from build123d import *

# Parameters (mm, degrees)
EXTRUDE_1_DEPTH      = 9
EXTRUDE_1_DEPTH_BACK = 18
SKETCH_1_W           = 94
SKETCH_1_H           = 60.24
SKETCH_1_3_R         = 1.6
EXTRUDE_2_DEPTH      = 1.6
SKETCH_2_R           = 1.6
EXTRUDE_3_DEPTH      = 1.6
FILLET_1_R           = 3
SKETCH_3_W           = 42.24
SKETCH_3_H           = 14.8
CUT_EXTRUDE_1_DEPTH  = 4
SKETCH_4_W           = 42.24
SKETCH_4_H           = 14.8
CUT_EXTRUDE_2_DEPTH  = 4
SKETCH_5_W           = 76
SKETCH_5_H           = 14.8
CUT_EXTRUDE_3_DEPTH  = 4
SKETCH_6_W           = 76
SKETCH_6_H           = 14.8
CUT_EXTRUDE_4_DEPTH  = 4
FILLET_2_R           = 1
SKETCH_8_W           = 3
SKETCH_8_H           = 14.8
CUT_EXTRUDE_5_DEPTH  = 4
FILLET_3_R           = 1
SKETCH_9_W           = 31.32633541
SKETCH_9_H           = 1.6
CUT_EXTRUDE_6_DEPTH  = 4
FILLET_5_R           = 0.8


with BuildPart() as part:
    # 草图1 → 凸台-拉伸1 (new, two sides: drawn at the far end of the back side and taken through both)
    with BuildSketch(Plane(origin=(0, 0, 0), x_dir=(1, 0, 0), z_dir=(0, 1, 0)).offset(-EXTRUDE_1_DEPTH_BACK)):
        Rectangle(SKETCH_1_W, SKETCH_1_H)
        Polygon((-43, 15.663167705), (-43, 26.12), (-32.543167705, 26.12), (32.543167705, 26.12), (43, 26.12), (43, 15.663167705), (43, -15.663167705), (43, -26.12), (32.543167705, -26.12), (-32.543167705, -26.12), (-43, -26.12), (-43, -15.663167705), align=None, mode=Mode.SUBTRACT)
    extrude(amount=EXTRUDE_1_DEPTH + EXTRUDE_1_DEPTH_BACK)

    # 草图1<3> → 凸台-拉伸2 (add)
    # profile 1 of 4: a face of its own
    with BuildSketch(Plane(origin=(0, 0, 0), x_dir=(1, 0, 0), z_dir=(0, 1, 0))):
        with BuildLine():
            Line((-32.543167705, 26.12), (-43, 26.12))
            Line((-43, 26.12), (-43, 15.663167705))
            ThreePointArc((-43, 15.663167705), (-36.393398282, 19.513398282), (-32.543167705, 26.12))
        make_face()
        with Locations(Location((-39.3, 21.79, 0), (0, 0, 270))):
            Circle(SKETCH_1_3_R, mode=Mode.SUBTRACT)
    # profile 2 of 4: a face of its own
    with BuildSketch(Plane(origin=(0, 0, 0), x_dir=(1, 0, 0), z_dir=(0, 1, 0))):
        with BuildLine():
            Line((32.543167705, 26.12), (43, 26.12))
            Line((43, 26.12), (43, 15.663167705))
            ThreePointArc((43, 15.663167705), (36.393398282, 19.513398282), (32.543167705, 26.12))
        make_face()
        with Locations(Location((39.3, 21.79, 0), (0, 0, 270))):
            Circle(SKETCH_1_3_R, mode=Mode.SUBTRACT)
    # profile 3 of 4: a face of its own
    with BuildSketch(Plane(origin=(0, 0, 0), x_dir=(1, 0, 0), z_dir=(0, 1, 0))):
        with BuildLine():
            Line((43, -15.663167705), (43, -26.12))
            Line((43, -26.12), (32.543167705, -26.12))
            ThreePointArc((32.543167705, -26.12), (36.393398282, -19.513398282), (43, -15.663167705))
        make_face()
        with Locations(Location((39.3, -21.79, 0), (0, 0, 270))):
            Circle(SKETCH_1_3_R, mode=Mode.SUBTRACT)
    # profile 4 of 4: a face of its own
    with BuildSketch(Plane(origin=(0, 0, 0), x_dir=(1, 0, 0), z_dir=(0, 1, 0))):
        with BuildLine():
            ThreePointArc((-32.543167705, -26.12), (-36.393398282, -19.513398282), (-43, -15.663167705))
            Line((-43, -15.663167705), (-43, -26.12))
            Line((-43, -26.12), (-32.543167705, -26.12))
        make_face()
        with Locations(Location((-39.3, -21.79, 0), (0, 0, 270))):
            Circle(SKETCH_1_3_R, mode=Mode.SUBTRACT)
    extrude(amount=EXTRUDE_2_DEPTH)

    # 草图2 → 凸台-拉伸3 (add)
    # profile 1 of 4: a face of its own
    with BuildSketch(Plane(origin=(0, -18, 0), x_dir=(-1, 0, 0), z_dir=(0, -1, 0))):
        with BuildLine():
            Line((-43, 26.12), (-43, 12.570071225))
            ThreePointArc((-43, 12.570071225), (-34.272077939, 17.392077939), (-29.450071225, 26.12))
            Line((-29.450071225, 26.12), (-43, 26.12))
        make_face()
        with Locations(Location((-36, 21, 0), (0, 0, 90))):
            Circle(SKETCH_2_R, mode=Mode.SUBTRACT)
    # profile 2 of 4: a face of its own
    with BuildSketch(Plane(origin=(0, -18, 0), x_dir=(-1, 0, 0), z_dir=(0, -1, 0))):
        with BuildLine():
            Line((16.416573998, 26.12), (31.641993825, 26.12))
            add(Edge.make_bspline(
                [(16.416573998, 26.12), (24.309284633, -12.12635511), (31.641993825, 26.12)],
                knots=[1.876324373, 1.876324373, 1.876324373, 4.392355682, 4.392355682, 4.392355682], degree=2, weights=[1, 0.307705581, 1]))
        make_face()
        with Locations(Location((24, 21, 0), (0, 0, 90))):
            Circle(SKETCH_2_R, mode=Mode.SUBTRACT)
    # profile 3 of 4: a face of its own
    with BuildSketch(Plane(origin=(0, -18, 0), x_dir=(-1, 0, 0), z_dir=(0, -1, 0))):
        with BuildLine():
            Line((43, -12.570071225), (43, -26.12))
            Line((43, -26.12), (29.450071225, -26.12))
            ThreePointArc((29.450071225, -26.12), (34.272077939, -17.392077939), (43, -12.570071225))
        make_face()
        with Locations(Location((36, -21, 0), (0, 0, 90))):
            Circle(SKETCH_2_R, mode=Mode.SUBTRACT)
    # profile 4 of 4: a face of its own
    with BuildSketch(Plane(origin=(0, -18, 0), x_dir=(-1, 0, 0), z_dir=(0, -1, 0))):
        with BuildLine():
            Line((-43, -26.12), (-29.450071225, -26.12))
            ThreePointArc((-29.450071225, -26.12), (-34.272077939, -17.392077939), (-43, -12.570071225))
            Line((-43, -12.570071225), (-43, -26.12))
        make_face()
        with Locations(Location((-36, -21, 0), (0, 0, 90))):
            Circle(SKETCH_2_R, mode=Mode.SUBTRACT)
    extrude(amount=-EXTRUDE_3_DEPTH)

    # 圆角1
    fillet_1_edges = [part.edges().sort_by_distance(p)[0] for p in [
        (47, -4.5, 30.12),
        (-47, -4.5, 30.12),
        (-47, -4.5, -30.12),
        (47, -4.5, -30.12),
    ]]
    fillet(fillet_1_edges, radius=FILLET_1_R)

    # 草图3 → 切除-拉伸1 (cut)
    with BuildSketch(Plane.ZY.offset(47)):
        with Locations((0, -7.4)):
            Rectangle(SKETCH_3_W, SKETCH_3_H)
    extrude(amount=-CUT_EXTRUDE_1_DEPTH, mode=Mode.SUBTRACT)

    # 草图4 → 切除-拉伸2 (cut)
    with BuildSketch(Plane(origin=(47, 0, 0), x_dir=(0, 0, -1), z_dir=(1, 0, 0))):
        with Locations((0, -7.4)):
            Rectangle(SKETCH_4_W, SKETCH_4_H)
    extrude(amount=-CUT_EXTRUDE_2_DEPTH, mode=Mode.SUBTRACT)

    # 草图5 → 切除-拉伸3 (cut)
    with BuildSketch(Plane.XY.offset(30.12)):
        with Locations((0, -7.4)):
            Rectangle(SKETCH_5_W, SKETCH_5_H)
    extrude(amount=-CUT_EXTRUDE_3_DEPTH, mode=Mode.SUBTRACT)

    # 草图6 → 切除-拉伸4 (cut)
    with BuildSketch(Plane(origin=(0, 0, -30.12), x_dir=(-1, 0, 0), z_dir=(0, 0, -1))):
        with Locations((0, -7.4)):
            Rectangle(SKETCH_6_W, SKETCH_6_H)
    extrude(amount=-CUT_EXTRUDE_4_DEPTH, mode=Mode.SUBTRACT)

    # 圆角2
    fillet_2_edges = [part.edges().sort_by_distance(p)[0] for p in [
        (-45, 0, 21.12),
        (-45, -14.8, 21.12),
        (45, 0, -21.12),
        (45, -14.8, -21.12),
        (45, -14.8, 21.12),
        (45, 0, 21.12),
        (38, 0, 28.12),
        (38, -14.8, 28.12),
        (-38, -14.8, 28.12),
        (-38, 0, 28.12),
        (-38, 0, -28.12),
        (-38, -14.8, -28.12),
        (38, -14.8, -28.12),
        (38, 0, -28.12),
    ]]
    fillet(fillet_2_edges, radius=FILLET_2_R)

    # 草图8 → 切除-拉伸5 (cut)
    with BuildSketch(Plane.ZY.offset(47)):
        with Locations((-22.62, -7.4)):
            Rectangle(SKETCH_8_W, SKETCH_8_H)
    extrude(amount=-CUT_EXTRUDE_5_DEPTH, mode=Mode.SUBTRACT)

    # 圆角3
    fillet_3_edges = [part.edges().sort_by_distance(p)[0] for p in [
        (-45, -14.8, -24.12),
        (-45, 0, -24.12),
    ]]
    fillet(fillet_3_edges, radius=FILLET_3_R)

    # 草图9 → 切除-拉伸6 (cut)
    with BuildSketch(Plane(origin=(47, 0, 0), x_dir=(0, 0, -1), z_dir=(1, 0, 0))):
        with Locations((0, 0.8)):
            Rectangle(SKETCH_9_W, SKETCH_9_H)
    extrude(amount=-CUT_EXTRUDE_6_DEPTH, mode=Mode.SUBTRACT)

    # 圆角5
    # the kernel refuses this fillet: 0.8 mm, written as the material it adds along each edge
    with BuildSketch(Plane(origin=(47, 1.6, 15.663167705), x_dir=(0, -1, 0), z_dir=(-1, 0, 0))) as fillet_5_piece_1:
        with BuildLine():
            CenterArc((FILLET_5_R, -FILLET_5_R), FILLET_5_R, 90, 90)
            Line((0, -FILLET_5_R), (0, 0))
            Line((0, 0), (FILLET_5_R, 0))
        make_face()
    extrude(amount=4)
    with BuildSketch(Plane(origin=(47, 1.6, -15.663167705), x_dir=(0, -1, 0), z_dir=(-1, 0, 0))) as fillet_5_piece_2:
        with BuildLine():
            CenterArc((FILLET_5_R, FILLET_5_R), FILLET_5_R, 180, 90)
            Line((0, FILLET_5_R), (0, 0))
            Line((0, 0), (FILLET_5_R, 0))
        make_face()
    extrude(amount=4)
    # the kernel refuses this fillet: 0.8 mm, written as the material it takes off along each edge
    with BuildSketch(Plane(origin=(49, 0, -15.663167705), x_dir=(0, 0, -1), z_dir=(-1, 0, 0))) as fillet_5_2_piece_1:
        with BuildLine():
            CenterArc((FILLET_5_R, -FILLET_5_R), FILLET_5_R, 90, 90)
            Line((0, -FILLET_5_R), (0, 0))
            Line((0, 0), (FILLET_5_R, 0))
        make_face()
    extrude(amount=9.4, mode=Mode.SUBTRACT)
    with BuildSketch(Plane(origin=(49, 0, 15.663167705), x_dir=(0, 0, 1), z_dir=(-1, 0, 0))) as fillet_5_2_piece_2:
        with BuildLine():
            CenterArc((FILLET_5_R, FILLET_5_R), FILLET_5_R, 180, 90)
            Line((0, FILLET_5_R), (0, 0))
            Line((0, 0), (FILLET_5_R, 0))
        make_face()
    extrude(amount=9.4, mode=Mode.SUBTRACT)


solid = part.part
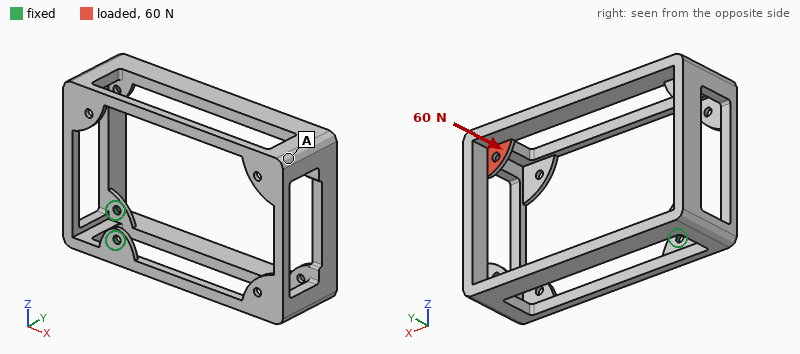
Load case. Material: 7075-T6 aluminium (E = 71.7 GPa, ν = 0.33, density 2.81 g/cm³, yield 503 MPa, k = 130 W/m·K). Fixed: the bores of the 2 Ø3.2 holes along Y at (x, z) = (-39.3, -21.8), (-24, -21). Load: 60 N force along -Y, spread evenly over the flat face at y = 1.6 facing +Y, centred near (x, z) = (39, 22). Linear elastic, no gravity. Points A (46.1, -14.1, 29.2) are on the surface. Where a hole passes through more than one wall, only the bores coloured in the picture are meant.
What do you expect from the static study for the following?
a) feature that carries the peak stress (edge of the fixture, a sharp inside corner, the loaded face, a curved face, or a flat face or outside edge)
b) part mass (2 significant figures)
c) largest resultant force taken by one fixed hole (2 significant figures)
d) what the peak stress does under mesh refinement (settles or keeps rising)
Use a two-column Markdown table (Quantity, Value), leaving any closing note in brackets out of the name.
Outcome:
| Quantity | Value |
|---|---|
| feature that carries the peak stress | edge of the fixture |
| part mass | 51 g |
| largest resultant force taken by one fixed hole | 280 N |
| what the peak stress does under mesh refinement | keeps rising |
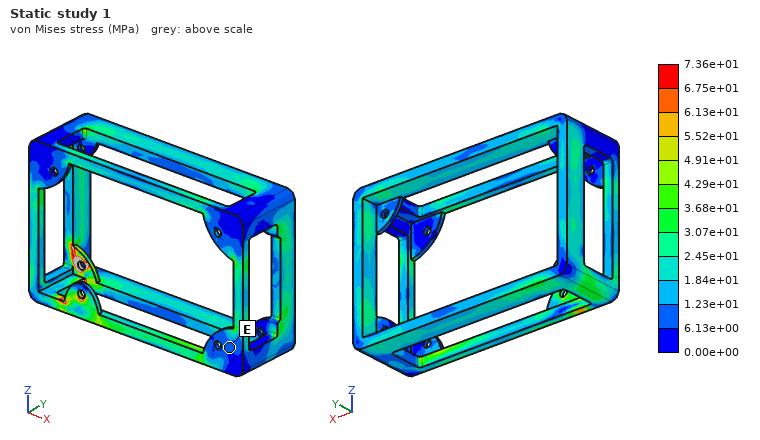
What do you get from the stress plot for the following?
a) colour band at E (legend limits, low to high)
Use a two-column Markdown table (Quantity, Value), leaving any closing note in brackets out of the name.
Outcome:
| Quantity | Value |
|---|---|
| colour band at E | 6.13e+00 to 1.23e+01 MPa |
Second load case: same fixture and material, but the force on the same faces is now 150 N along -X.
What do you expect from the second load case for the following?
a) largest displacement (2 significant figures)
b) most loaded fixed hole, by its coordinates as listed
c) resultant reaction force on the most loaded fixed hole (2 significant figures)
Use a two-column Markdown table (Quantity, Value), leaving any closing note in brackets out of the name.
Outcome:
| Quantity | Value |
|---|---|
| largest displacement | 1.3 mm |
| most loaded fixed hole, by its coordinates as listed | (-39.3, -21.8) |
| resultant reaction force on the most loaded fixed hole | 170 N |
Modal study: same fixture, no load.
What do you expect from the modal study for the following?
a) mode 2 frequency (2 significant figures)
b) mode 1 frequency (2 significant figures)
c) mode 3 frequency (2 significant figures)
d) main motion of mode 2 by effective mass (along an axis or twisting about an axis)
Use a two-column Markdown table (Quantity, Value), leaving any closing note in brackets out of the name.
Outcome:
| Quantity | Value |
|---|---|
| mode 2 frequency | 360 Hz |
| mode 1 frequency | 250 Hz |
| mode 3 frequency | 740 Hz |
| main motion of mode 2 by effective mass | along Y |
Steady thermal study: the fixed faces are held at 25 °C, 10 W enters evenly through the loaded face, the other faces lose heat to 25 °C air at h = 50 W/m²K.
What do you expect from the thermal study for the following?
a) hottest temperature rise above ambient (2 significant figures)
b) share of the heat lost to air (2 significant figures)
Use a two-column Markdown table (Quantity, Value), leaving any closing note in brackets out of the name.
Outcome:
| Quantity | Value |
|---|---|
| hottest temperature rise above ambient | 48 K |
| share of the heat lost to air | 88 % |
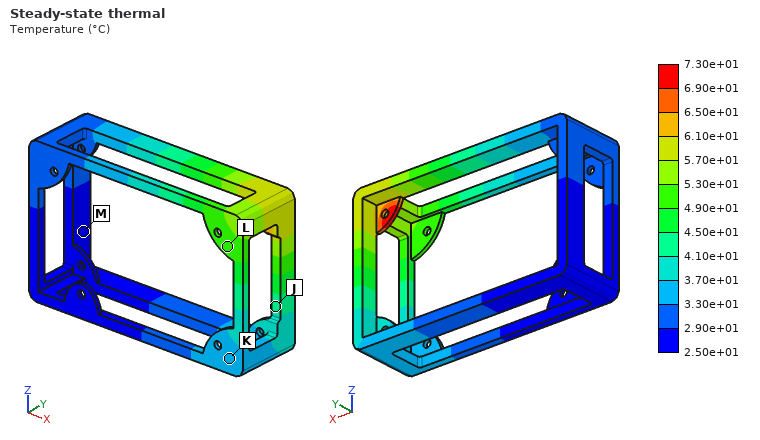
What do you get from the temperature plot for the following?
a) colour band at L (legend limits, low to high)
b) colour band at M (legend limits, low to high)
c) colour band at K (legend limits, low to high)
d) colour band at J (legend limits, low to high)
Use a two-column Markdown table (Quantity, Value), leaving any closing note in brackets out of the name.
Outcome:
| Quantity | Value |
|---|---|
| colour band at L | 4.90e+01 to 5.30e+01 °C |
| colour band at M | 2.50e+01 to 2.90e+01 °C |
| colour band at K | 3.30e+01 to 3.70e+01 °C |
| colour band at J | 4.10e+01 to 4.50e+01 °C |
